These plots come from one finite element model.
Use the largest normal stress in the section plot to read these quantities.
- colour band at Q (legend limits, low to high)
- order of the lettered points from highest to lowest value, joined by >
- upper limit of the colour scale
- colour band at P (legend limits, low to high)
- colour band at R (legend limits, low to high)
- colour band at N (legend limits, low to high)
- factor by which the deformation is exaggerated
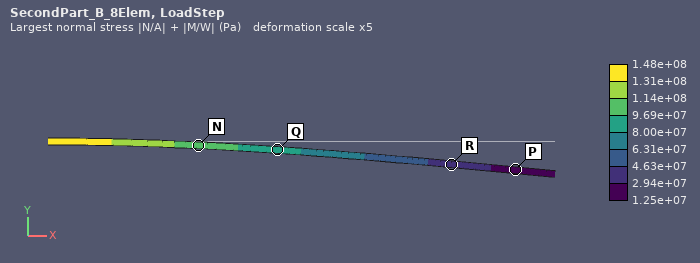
8.00e+07 to 9.69e+07 Pa
N > Q > R > P
1.48e+08 Pa
1.25e+07 to 2.94e+07 Pa
2.94e+07 to 4.63e+07 Pa
9.69e+07 to 1.14e+08 Pa
5
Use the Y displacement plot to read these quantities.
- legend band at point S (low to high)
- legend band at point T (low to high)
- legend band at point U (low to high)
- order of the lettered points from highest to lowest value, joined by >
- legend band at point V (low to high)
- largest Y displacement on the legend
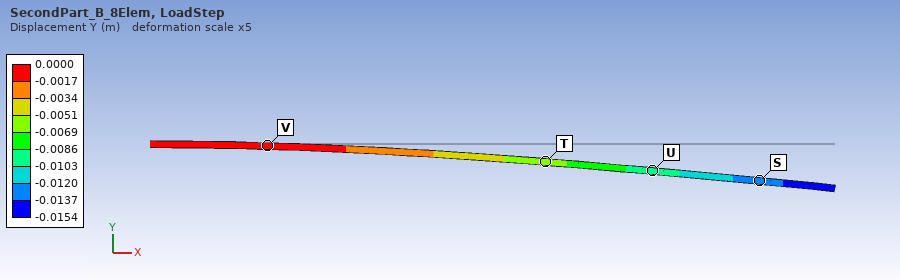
-0.0137 to -0.0120 m
-0.0069 to -0.0051 m
-0.0103 to -0.0086 m
V > T > U > S
-0.0017 to 0.0000 m
0.0000 m
